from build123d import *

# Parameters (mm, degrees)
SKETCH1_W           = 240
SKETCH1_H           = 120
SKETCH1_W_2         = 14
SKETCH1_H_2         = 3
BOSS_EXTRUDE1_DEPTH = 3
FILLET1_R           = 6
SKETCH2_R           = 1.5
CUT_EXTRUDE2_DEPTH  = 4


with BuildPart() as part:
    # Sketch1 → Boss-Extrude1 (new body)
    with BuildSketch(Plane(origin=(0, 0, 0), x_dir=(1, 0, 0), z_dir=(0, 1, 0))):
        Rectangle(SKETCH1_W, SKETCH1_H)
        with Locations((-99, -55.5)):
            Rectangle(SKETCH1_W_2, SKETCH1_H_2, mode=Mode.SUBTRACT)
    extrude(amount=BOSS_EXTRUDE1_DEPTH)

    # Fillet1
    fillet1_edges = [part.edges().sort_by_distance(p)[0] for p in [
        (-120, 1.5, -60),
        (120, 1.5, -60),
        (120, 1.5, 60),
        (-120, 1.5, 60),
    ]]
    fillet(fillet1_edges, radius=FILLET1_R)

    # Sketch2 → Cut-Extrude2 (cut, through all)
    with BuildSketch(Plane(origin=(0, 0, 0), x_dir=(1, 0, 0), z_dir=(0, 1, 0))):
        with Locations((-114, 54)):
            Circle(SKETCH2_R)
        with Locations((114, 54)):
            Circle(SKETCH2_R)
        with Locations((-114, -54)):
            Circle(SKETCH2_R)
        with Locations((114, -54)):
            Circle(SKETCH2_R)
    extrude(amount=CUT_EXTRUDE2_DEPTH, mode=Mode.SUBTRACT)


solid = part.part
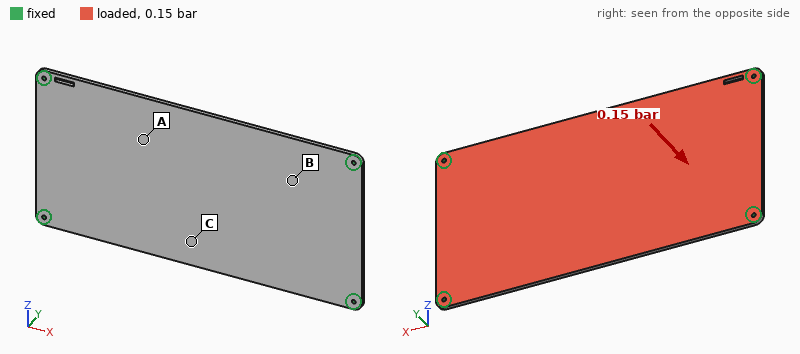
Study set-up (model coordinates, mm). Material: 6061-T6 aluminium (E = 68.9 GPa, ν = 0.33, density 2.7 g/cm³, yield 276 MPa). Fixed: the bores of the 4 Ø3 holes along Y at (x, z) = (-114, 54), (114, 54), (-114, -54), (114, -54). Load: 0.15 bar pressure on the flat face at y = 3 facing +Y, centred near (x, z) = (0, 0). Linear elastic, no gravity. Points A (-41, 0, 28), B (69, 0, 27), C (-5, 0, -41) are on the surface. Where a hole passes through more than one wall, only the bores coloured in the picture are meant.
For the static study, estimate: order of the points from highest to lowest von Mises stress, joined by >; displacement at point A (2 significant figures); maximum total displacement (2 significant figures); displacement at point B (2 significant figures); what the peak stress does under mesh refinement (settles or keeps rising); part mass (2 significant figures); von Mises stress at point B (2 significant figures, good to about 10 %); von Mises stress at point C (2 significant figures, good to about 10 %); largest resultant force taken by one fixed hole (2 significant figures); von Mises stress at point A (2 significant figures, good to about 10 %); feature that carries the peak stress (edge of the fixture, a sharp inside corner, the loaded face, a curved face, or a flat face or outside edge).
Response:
C > A > B
0.89 mm
1.1 mm
0.57 mm
keeps rising
230 g
9.1 MPa
28 MPa
110 N
19 MPa
edge of the fixture
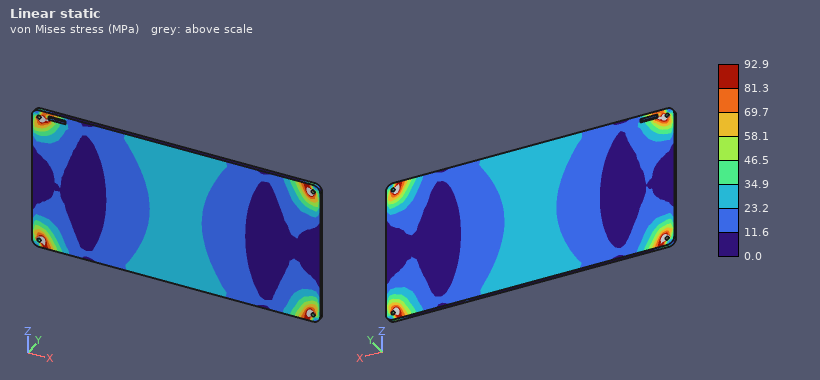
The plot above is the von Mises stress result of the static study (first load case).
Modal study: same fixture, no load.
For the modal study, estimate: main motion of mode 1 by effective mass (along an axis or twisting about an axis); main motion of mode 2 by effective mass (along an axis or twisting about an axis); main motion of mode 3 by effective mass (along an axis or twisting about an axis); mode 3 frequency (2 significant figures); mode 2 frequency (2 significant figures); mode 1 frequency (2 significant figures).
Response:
along Y
twisting about X
twisting about Z
670 Hz
460 Hz
230 Hz
